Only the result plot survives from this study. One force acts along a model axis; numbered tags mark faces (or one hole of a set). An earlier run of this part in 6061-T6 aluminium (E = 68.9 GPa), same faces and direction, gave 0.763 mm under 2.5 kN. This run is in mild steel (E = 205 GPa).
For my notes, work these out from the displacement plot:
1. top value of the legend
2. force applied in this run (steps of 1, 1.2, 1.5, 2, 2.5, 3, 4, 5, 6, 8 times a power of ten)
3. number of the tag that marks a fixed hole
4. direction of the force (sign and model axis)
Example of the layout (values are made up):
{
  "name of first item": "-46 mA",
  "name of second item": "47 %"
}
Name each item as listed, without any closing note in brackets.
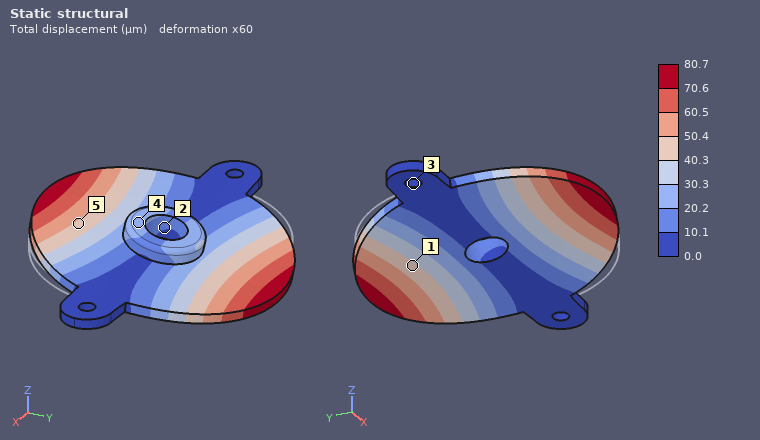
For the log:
{
  "top value of the legend": "80.7 µm",
  "force applied in this run": "800 N",
  "number of the tag that marks a fixed hole": "3",
  "direction of the force": "+Y"
}
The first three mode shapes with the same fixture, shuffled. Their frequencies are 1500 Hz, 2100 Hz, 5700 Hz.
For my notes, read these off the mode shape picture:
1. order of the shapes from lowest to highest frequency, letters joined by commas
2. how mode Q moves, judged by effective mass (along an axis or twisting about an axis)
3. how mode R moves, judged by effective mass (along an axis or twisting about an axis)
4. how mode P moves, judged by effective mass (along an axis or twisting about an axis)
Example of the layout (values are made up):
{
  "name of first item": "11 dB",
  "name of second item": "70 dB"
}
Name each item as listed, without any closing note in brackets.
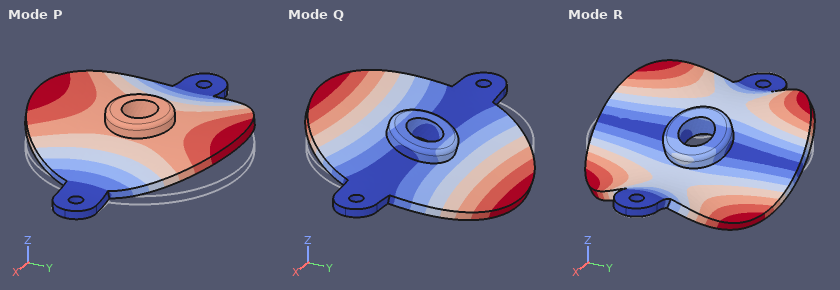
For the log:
{
  "order of the shapes from lowest to highest frequency, letters joined by commas": "Q, P, R",
  "how mode Q moves, judged by effective mass": "twisting about X",
  "how mode R moves, judged by effective mass": "twisting about Y",
  "how mode P moves, judged by effective mass": "along Z"
}
